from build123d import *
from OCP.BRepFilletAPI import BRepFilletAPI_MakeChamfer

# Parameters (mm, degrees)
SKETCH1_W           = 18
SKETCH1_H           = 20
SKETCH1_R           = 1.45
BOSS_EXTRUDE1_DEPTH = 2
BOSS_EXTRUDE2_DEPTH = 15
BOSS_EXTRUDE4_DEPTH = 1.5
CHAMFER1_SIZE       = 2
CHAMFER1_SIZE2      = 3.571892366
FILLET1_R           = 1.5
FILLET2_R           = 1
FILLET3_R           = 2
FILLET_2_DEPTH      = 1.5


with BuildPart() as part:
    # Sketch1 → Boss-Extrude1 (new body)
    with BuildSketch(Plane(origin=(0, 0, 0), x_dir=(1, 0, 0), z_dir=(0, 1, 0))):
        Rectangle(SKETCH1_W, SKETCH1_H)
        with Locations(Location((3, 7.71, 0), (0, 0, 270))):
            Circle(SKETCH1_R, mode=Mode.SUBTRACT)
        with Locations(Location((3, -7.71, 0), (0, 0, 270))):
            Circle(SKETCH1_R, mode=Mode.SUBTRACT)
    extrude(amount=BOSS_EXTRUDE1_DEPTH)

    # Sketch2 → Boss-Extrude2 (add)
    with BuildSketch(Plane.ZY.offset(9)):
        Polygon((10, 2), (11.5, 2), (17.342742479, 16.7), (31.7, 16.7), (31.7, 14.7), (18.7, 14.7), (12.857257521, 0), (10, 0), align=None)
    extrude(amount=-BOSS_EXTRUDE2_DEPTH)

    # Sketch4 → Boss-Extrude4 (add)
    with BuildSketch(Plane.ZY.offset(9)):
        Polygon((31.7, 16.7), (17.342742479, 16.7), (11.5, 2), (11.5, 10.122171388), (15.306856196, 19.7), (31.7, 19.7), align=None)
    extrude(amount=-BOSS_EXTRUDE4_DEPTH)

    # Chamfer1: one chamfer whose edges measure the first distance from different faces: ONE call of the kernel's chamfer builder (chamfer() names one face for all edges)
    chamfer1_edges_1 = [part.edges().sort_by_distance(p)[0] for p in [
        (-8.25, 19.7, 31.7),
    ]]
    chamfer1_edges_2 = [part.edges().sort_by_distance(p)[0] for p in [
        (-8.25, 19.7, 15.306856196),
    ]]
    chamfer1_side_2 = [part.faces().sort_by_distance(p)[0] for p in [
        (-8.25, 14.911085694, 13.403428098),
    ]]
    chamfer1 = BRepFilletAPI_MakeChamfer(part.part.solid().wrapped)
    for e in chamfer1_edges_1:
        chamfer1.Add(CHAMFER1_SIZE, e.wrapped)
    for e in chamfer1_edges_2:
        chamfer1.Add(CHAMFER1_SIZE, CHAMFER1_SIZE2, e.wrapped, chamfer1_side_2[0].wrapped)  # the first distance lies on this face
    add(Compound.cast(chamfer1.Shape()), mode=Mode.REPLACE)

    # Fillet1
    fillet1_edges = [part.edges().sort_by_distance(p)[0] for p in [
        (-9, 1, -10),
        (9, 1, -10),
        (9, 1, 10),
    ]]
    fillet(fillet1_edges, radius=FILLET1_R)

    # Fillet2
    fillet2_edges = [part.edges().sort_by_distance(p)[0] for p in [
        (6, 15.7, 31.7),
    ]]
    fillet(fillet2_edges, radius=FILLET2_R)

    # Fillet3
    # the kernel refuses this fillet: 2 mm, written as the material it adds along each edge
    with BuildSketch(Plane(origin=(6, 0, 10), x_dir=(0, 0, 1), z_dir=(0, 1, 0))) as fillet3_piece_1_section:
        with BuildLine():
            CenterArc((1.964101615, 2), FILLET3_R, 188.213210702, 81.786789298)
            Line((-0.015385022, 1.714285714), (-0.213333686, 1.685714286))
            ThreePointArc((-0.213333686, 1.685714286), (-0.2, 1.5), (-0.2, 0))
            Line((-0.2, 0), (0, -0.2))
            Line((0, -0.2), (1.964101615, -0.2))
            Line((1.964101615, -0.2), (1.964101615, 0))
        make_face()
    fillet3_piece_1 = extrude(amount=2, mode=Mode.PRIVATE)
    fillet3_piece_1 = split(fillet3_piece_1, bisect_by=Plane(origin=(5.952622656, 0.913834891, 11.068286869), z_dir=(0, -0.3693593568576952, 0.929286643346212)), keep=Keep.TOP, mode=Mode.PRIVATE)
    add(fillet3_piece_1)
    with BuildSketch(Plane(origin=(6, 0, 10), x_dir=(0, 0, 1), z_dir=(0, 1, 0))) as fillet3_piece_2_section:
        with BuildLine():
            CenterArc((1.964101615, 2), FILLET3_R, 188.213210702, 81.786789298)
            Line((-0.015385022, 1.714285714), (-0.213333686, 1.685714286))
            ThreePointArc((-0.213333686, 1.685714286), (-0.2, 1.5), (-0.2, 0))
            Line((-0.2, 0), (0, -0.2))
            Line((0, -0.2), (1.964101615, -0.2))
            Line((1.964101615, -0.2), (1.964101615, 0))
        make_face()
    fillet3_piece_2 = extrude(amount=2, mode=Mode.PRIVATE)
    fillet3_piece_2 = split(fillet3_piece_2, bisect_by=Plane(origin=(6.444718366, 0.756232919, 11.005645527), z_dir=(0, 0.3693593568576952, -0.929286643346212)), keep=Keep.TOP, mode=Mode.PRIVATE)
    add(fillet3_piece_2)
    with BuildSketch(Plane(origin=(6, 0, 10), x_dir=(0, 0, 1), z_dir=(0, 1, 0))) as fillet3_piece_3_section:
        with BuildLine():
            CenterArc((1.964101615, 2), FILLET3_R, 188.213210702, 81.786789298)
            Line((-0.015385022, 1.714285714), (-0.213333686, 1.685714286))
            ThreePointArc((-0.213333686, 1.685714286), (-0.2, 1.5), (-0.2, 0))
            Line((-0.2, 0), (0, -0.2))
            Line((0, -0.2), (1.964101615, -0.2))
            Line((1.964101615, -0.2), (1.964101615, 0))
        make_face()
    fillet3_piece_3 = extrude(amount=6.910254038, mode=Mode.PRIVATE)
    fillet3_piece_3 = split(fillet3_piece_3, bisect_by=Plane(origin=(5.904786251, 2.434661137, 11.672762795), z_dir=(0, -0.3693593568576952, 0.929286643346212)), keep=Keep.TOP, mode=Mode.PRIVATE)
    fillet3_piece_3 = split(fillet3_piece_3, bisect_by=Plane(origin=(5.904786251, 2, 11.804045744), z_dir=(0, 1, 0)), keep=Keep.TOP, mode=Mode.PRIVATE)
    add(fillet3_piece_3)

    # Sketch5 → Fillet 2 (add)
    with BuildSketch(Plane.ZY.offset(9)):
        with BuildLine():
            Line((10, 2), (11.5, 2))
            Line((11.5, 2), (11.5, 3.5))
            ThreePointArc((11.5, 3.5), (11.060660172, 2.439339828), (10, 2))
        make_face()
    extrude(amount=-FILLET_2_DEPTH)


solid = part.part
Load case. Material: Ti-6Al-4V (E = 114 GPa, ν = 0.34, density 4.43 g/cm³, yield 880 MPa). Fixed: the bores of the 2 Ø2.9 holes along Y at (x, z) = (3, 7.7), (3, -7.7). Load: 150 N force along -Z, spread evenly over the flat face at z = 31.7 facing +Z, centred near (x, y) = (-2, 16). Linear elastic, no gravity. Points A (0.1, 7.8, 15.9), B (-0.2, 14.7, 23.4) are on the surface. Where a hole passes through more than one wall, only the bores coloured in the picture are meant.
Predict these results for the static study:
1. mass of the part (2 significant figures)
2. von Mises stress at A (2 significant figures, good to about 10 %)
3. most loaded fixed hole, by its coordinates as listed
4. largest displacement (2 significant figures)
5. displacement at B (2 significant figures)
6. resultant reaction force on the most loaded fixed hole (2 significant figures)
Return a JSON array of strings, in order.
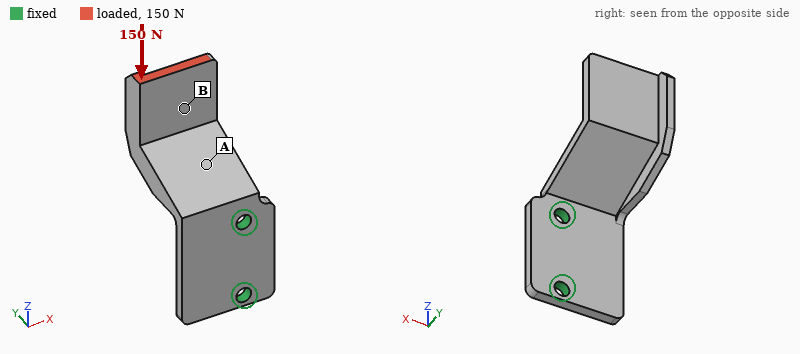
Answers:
["7.8 g", "73 MPa", "(3, 7.7)", "0.49 mm", "0.31 mm", "130 N"]
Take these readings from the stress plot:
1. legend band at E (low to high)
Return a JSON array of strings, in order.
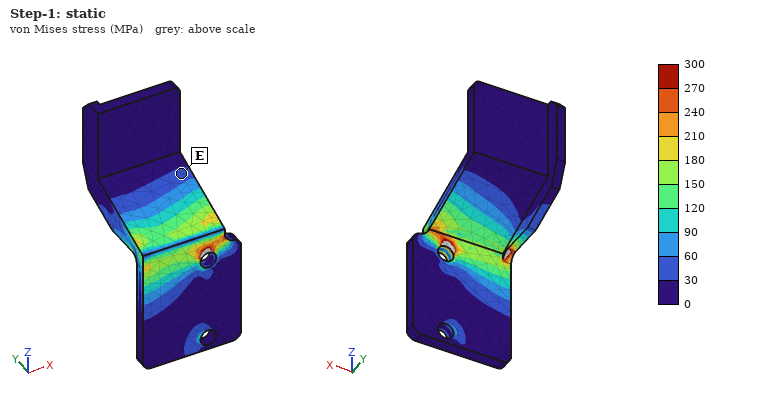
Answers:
["30 to 60 MPa"]
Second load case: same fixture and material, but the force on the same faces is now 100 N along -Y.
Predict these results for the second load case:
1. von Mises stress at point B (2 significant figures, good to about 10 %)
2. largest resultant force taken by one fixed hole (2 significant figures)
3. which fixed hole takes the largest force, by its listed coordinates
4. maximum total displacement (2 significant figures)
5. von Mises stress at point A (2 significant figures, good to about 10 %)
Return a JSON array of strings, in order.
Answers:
["41 MPa", "150 N", "(3, 7.7)", "0.58 mm", "100 MPa"]
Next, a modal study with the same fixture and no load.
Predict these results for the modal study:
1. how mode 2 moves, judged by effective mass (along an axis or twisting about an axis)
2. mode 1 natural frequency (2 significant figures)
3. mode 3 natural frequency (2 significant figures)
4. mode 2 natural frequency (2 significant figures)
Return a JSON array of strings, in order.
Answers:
["along X", "1600 Hz", "5200 Hz", "3500 Hz"]
